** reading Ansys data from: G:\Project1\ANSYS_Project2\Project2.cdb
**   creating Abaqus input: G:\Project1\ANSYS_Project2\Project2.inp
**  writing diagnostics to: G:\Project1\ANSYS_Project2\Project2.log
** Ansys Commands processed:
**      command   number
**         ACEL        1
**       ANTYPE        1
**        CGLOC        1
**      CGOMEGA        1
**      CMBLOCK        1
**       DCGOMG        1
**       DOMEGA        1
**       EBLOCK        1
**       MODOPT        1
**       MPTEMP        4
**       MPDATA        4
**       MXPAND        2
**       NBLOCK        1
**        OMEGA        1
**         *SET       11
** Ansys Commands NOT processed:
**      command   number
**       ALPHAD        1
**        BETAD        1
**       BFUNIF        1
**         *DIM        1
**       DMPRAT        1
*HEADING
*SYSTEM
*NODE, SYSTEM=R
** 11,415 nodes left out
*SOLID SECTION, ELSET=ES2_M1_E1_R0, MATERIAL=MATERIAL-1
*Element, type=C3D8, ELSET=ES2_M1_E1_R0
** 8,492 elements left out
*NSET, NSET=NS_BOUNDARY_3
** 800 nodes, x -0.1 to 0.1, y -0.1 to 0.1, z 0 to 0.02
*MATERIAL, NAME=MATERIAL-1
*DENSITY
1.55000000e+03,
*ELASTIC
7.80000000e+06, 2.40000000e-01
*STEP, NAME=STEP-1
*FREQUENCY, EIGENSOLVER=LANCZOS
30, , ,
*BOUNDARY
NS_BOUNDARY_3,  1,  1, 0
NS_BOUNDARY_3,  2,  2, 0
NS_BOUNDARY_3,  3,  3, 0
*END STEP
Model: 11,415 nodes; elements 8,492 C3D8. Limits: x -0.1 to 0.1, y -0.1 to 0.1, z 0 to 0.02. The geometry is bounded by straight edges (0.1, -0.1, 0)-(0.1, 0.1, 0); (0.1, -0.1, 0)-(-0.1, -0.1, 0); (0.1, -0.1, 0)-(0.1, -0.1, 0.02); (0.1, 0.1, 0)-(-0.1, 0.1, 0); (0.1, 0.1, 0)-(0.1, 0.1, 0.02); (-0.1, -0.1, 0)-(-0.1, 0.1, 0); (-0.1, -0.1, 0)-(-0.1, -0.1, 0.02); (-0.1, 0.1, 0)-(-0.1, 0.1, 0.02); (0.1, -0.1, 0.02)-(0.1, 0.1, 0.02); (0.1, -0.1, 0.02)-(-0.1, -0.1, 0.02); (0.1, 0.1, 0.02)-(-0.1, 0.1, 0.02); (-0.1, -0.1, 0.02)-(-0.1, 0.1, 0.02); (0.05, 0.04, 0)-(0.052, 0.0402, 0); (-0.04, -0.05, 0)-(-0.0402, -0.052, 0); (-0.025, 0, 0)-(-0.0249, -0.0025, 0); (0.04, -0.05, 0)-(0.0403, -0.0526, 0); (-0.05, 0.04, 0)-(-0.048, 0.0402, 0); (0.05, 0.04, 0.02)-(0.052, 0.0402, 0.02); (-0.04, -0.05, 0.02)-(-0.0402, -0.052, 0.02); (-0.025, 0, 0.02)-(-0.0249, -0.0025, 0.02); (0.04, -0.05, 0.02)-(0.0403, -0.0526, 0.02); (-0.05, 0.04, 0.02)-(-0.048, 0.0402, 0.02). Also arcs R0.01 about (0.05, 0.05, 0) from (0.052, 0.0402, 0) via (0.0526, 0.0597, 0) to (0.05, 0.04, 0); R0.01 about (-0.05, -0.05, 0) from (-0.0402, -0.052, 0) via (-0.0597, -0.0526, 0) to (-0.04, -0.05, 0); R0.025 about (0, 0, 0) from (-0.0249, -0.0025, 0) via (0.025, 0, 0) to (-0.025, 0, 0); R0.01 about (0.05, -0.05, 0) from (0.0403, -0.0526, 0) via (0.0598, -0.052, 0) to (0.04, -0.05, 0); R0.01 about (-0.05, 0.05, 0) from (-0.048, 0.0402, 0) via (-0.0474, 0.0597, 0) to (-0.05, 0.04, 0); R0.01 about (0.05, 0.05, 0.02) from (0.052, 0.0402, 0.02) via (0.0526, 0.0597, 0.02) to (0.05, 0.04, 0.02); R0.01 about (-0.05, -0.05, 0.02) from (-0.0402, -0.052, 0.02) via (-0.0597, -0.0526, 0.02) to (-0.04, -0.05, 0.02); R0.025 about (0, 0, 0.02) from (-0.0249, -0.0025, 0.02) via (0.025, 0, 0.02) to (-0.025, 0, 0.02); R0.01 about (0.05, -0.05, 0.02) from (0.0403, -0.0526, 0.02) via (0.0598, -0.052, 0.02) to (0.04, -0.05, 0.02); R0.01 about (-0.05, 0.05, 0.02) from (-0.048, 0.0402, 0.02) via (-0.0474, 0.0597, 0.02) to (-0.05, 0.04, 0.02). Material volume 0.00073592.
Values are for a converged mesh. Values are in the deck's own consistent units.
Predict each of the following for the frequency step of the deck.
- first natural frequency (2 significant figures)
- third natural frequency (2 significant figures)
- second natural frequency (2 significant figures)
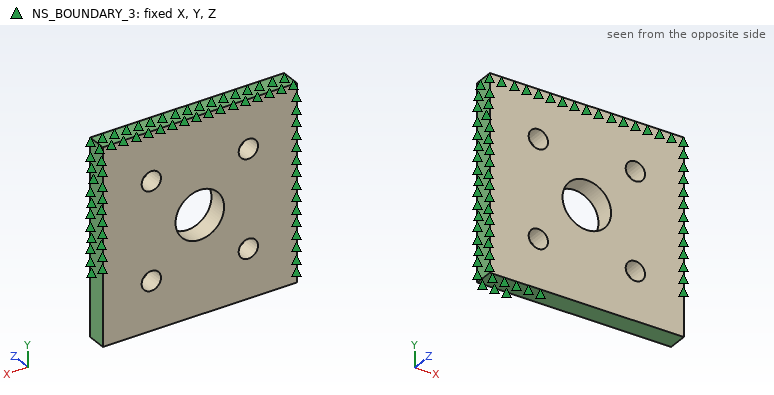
58 cycles per unit time
99 cycles per unit time
99 cycles per unit time
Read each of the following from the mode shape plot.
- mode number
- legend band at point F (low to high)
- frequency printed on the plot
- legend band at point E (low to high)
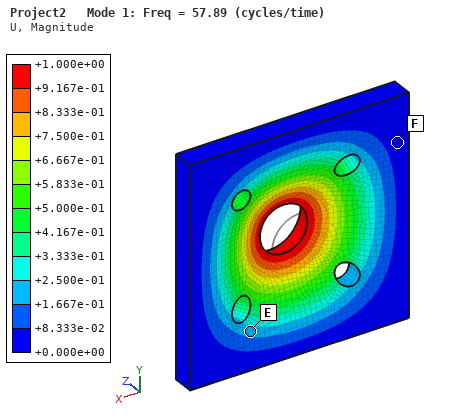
1
+0.000e+00 to +8.333e-02
57.89
+1.667e-01 to +2.500e-01
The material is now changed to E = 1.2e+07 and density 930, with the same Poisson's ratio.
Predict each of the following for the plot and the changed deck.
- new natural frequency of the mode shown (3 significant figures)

92.7
